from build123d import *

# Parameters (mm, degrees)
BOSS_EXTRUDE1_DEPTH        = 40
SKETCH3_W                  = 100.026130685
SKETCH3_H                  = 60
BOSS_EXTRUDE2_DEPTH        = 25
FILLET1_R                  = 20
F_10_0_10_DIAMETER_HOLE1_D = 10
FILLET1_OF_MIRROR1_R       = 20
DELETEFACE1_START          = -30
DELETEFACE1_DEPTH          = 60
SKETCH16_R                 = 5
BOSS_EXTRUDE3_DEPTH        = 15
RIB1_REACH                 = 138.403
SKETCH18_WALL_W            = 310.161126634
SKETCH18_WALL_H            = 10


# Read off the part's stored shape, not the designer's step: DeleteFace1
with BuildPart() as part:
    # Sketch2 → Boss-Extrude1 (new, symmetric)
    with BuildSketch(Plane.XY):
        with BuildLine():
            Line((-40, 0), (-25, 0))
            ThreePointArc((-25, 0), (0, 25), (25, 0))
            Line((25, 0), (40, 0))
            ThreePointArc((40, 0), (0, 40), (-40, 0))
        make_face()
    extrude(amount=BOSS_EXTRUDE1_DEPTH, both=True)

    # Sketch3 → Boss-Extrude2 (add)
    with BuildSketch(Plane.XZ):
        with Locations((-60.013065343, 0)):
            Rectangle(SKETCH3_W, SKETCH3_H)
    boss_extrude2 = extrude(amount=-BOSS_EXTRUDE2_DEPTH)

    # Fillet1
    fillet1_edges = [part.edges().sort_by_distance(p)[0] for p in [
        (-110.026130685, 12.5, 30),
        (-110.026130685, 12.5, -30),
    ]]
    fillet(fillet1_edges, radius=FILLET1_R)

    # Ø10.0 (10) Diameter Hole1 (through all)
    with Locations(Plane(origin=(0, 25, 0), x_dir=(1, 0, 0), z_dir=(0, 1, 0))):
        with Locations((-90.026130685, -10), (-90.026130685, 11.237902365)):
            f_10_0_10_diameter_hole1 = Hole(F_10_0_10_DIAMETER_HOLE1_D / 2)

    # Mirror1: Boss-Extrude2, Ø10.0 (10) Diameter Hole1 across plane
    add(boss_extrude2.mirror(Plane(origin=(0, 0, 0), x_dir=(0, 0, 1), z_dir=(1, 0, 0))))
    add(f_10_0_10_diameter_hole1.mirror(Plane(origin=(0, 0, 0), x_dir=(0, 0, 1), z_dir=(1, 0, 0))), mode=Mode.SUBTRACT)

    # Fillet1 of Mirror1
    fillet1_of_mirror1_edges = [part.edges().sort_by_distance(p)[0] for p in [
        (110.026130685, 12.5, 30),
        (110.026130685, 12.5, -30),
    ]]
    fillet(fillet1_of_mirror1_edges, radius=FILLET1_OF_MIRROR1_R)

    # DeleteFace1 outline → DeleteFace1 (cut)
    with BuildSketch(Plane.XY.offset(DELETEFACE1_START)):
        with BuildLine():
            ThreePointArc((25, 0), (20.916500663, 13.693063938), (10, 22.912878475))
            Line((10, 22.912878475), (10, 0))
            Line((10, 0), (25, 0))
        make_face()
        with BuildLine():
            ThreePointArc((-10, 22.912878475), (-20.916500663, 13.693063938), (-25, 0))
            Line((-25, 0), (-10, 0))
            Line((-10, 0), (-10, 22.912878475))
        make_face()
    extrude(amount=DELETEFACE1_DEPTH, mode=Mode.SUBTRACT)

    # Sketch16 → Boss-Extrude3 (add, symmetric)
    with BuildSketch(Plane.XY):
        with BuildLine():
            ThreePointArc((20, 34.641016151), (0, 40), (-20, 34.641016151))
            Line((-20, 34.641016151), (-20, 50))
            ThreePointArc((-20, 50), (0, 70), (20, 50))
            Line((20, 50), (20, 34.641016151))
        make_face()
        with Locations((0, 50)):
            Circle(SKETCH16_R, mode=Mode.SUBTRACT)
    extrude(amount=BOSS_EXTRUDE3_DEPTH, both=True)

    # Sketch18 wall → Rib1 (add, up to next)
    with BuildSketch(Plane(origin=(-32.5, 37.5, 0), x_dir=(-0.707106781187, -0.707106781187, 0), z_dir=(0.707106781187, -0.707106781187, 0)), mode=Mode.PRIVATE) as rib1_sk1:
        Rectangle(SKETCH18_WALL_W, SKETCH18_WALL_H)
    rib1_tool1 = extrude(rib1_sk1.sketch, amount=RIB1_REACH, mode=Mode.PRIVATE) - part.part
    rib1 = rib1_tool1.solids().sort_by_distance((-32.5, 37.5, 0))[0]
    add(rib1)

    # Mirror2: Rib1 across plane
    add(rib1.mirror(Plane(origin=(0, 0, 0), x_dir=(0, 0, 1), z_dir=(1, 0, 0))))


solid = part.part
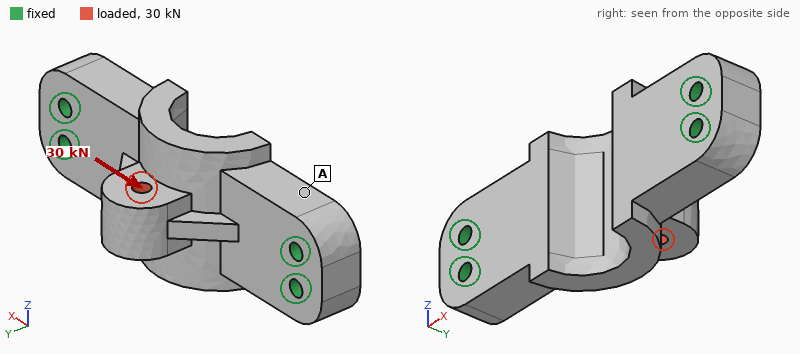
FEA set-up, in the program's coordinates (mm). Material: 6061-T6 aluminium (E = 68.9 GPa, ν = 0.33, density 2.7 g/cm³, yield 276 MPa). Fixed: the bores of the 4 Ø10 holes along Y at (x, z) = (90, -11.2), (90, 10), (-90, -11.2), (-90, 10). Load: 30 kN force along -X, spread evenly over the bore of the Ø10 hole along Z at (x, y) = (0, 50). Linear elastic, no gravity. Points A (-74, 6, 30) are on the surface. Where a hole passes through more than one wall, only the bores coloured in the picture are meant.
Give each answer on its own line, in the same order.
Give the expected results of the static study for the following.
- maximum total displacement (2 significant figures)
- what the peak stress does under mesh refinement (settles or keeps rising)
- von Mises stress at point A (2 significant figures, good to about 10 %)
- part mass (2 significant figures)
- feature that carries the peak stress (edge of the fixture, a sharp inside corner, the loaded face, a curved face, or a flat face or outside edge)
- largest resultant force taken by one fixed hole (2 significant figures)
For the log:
0.11 mm
keeps rising
13 MPa
970 g
edge of the fixture
9.0 kN
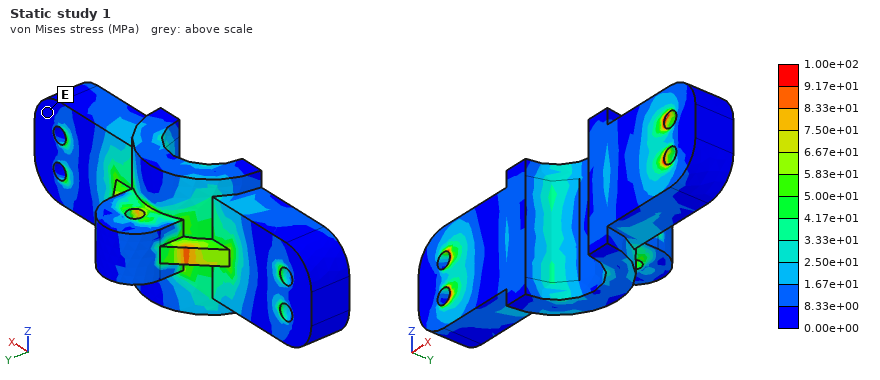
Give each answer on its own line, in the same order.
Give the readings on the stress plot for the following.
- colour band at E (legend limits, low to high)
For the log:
0.00e+00 to 8.33e+00 MPa
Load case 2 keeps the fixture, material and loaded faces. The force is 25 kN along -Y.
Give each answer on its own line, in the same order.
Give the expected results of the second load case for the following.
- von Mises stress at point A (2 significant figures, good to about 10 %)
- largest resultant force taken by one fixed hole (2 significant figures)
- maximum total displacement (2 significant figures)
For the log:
23 MPa
12 kN
0.12 mm
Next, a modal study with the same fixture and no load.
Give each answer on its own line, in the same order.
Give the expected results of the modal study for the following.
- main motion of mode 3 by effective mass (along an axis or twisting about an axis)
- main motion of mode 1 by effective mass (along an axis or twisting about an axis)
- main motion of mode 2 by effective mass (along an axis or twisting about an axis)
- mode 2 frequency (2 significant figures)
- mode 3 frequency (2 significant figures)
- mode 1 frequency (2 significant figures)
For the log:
along Z
along Z
along Y
3500 Hz
6000 Hz
3100 Hz
